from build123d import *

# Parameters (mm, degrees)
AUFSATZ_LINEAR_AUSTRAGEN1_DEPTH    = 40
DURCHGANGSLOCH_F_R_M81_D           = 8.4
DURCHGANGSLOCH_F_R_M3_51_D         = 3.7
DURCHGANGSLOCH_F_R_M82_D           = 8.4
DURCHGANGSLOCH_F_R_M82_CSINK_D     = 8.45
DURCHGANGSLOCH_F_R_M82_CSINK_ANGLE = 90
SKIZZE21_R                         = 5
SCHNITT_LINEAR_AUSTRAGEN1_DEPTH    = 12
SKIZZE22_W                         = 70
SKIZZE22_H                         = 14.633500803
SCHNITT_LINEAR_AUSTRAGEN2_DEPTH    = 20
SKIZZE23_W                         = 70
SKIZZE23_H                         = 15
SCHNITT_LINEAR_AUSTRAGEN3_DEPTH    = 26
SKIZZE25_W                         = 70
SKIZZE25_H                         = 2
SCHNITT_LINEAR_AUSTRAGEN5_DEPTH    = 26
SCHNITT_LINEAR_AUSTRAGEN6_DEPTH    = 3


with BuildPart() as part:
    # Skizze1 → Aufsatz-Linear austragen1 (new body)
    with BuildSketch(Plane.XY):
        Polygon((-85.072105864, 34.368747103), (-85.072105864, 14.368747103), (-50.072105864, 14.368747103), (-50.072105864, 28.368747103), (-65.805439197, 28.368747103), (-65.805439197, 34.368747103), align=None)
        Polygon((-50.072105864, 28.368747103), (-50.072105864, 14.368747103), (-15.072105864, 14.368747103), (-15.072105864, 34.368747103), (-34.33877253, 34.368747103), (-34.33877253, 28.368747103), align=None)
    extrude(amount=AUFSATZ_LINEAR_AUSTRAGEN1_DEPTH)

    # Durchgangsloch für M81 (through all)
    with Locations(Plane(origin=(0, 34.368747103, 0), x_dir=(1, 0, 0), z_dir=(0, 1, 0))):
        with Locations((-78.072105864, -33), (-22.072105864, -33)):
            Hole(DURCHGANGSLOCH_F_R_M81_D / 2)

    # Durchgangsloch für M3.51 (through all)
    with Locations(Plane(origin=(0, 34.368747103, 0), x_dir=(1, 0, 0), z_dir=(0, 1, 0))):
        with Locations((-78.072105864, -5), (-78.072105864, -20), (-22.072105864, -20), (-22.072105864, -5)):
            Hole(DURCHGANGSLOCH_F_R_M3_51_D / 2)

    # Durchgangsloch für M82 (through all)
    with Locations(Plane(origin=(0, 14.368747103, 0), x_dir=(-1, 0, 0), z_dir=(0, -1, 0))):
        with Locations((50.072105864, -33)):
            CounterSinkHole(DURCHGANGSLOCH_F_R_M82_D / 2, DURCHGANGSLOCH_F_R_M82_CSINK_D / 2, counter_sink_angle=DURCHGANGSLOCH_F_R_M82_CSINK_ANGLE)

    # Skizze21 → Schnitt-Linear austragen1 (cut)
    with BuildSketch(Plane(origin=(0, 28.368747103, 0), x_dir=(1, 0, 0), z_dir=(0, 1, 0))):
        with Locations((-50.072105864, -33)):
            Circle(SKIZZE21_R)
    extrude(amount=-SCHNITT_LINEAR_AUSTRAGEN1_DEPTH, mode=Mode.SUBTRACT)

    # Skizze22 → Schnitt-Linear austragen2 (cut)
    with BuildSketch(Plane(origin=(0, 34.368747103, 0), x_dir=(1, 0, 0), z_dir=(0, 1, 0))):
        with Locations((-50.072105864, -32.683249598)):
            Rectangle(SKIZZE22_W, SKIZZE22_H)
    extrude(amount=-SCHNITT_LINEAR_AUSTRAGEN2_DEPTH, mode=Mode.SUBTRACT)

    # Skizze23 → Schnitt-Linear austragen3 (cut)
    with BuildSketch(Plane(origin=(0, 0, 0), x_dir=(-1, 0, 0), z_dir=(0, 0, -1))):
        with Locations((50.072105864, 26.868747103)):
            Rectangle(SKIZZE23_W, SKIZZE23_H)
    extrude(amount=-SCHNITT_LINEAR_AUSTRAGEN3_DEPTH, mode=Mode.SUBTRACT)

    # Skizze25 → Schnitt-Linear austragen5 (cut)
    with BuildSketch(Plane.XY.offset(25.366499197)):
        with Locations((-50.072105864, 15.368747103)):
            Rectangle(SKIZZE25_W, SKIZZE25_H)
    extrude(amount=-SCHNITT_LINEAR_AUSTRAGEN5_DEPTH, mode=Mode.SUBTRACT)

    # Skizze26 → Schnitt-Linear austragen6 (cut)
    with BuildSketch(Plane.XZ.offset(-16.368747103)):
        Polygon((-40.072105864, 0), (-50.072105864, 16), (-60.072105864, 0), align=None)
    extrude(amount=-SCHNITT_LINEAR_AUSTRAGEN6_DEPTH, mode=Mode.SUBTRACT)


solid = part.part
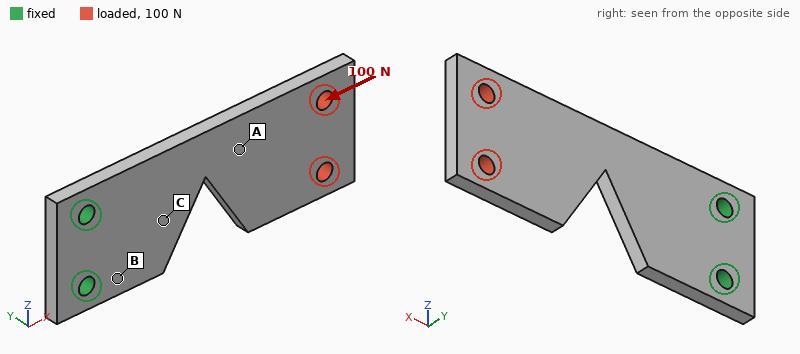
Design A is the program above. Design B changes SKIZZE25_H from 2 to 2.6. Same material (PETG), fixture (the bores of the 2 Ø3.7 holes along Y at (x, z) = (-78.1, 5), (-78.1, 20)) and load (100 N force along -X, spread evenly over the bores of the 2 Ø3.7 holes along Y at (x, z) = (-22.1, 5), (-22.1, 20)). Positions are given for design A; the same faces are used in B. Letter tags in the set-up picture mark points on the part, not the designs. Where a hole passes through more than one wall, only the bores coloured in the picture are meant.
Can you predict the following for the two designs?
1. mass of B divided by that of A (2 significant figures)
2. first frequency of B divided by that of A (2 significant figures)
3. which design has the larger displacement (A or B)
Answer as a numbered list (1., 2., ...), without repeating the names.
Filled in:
1. 0.90
2. 0.90
3. B
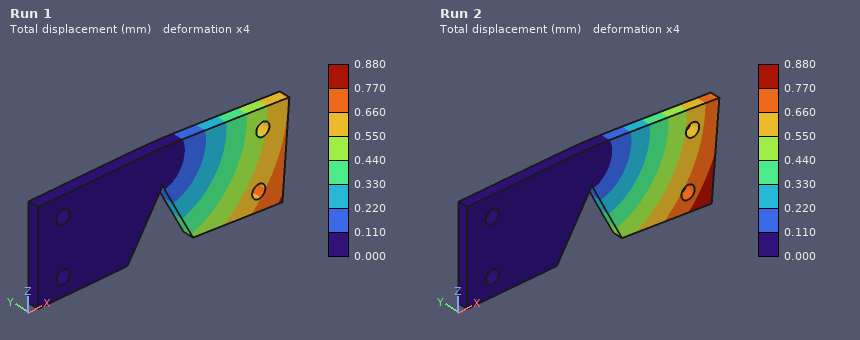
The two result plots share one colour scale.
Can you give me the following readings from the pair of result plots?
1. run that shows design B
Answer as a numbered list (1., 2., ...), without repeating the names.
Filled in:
1. Run 2
